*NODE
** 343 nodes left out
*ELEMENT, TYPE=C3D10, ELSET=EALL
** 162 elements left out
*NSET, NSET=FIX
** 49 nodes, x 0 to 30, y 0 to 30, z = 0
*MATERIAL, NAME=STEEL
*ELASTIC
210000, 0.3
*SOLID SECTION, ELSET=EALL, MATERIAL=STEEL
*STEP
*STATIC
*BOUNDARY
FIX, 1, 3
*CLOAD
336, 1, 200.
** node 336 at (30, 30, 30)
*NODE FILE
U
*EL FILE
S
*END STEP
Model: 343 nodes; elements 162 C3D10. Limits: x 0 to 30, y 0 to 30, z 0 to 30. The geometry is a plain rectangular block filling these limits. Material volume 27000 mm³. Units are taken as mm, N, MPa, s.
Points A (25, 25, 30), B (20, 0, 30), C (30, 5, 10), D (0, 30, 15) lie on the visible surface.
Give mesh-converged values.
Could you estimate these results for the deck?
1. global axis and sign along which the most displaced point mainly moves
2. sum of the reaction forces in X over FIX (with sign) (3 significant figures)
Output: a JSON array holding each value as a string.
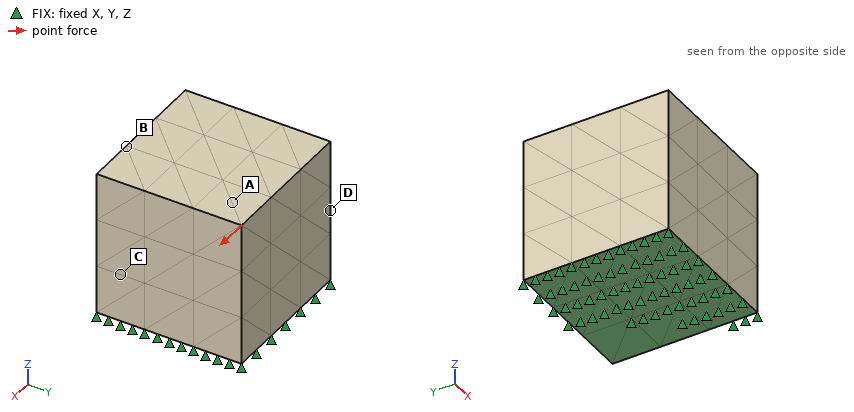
["+X", "-200 N"]
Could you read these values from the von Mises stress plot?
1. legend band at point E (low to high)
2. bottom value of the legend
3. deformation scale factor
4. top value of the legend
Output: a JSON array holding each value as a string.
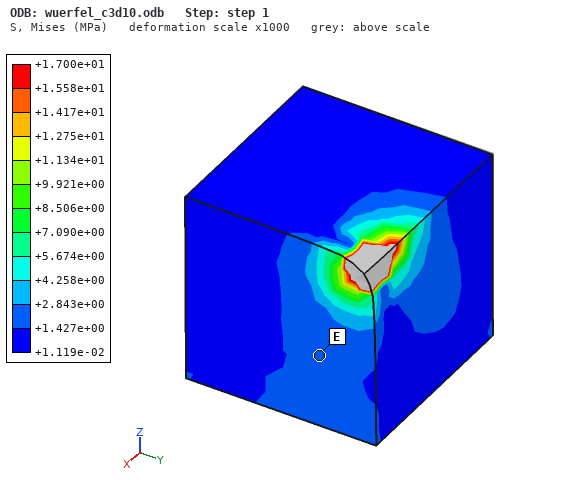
["+1.427e+00 to +2.843e+00 MPa", "+1.119e-02 MPa", "1000", "+1.700e+01 MPa"]
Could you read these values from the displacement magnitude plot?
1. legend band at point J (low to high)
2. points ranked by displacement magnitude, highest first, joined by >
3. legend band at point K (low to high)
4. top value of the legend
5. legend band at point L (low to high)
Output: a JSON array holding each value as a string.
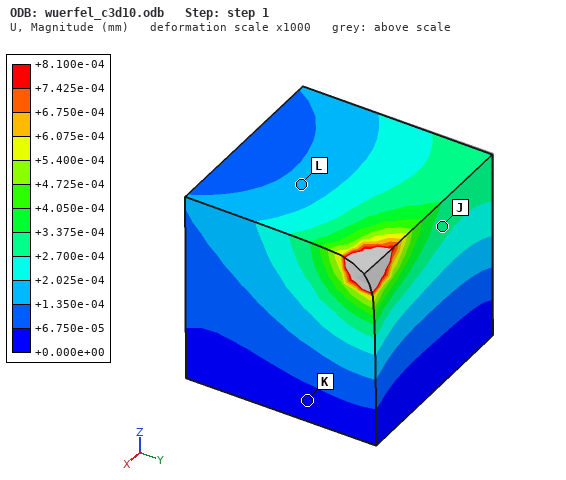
["+2.700e-04 to +3.375e-04 mm", "J > L > K", "+0.000e+00 to +6.750e-05 mm", "+8.100e-04 mm", "+1.350e-04 to +2.025e-04 mm"]
